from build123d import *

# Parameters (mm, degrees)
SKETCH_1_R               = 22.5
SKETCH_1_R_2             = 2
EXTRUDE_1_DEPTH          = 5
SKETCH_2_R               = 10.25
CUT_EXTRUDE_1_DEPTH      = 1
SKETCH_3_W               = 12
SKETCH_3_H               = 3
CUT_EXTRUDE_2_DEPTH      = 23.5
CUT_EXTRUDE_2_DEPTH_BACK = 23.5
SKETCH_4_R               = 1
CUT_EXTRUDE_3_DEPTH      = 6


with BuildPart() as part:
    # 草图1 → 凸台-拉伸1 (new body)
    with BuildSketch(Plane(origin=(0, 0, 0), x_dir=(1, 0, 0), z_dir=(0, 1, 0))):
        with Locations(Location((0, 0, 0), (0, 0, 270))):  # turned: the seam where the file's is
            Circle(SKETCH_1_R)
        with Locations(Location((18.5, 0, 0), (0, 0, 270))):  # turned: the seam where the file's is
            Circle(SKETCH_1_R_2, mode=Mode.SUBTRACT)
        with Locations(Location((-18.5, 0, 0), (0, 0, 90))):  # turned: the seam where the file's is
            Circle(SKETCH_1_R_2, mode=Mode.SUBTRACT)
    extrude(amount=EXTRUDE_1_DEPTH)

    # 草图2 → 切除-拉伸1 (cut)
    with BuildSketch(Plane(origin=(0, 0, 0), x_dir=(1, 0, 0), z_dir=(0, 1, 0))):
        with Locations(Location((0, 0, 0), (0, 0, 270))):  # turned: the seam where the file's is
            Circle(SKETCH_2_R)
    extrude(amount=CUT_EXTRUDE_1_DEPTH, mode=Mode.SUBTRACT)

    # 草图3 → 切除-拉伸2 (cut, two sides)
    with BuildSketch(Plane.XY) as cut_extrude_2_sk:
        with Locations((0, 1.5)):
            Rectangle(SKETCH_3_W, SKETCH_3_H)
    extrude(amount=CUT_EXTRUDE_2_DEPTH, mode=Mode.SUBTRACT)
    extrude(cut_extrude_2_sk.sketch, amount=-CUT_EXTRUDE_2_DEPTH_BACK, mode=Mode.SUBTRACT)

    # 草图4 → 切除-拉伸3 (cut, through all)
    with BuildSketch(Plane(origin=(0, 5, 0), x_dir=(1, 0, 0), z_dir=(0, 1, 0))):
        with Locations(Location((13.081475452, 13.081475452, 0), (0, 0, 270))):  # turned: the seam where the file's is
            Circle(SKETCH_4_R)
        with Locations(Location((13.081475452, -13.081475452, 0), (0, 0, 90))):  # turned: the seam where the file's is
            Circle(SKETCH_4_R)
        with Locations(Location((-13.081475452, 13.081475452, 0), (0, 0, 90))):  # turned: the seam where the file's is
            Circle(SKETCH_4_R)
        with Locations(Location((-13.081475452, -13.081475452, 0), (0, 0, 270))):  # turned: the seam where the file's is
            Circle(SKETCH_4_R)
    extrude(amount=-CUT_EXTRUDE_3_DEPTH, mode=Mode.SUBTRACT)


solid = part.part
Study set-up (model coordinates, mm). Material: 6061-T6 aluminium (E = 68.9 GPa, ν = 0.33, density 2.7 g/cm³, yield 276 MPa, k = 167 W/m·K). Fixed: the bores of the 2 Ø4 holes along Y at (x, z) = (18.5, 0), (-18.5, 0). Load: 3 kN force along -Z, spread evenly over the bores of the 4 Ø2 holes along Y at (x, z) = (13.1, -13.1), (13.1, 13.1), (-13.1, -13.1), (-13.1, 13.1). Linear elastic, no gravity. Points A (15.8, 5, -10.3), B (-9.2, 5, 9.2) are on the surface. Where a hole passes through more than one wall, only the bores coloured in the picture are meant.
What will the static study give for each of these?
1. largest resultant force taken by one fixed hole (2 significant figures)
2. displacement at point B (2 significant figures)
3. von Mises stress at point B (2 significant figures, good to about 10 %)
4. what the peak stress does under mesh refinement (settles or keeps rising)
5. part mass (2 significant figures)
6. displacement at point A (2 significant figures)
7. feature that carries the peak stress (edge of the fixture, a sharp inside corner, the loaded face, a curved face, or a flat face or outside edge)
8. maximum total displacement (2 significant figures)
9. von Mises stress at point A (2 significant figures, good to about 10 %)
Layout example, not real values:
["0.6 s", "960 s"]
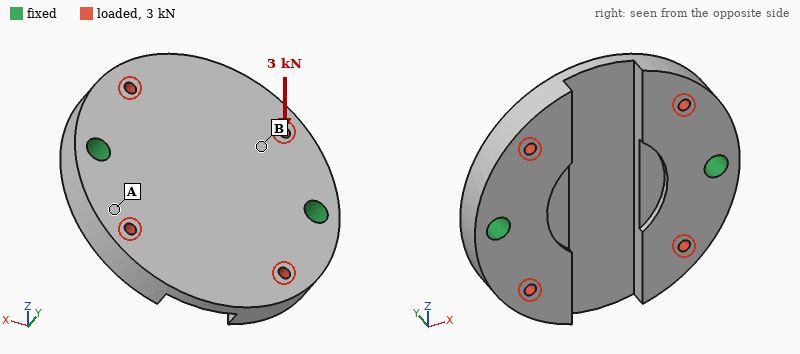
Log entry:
["1.5 kN", "5.1 µm", "7.5 MPa", "keeps rising", "16 g", "3.3 µm", "edge of the fixture", "7.6 µm", "21 MPa"]
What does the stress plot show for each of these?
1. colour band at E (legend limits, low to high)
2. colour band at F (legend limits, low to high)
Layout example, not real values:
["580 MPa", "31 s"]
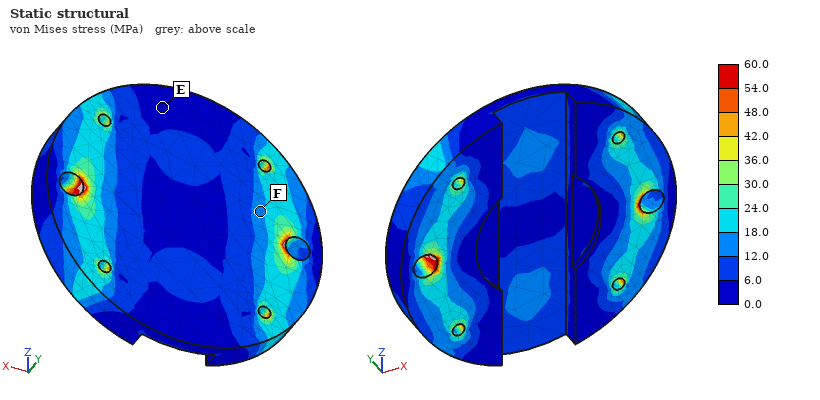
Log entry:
["0.0 to 6.0 MPa", "12.0 to 18.0 MPa"]
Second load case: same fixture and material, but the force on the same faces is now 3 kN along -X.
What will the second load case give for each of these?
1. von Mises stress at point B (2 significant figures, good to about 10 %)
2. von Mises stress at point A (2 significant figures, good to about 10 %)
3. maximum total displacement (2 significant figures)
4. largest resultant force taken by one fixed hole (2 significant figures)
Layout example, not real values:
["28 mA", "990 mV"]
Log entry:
["16 MPa", "17 MPa", "9.7 µm", "1.5 kN"]
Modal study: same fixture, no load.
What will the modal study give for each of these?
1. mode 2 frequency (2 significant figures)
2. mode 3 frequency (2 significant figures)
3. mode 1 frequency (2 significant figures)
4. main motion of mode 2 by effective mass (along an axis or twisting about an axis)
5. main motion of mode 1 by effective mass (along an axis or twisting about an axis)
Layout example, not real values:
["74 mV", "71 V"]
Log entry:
["9500 Hz", "14 kHz", "7500 Hz", "along Y", "twisting about X"]
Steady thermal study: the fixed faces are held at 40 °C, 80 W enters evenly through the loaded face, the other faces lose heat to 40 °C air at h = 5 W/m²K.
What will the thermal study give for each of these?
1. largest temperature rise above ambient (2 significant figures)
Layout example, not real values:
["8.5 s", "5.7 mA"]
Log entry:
["32 K"]
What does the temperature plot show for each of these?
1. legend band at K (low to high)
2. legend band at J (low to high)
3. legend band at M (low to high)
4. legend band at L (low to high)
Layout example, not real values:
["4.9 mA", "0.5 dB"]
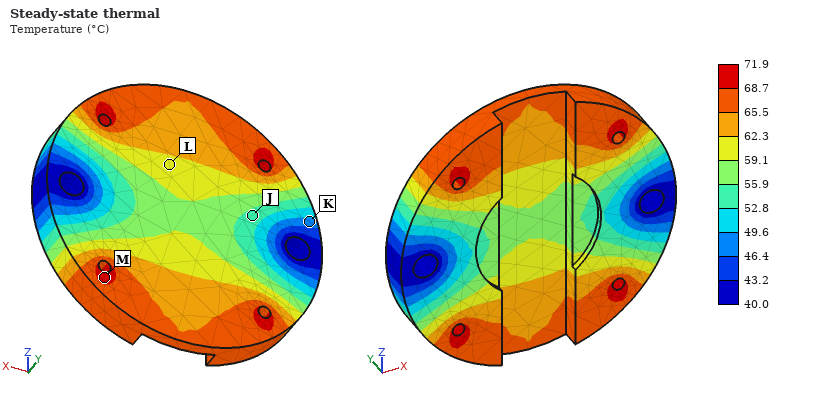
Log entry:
["46.4 to 49.6 °C", "52.8 to 55.9 °C", "68.7 to 71.9 °C", "59.1 to 62.3 °C"]
